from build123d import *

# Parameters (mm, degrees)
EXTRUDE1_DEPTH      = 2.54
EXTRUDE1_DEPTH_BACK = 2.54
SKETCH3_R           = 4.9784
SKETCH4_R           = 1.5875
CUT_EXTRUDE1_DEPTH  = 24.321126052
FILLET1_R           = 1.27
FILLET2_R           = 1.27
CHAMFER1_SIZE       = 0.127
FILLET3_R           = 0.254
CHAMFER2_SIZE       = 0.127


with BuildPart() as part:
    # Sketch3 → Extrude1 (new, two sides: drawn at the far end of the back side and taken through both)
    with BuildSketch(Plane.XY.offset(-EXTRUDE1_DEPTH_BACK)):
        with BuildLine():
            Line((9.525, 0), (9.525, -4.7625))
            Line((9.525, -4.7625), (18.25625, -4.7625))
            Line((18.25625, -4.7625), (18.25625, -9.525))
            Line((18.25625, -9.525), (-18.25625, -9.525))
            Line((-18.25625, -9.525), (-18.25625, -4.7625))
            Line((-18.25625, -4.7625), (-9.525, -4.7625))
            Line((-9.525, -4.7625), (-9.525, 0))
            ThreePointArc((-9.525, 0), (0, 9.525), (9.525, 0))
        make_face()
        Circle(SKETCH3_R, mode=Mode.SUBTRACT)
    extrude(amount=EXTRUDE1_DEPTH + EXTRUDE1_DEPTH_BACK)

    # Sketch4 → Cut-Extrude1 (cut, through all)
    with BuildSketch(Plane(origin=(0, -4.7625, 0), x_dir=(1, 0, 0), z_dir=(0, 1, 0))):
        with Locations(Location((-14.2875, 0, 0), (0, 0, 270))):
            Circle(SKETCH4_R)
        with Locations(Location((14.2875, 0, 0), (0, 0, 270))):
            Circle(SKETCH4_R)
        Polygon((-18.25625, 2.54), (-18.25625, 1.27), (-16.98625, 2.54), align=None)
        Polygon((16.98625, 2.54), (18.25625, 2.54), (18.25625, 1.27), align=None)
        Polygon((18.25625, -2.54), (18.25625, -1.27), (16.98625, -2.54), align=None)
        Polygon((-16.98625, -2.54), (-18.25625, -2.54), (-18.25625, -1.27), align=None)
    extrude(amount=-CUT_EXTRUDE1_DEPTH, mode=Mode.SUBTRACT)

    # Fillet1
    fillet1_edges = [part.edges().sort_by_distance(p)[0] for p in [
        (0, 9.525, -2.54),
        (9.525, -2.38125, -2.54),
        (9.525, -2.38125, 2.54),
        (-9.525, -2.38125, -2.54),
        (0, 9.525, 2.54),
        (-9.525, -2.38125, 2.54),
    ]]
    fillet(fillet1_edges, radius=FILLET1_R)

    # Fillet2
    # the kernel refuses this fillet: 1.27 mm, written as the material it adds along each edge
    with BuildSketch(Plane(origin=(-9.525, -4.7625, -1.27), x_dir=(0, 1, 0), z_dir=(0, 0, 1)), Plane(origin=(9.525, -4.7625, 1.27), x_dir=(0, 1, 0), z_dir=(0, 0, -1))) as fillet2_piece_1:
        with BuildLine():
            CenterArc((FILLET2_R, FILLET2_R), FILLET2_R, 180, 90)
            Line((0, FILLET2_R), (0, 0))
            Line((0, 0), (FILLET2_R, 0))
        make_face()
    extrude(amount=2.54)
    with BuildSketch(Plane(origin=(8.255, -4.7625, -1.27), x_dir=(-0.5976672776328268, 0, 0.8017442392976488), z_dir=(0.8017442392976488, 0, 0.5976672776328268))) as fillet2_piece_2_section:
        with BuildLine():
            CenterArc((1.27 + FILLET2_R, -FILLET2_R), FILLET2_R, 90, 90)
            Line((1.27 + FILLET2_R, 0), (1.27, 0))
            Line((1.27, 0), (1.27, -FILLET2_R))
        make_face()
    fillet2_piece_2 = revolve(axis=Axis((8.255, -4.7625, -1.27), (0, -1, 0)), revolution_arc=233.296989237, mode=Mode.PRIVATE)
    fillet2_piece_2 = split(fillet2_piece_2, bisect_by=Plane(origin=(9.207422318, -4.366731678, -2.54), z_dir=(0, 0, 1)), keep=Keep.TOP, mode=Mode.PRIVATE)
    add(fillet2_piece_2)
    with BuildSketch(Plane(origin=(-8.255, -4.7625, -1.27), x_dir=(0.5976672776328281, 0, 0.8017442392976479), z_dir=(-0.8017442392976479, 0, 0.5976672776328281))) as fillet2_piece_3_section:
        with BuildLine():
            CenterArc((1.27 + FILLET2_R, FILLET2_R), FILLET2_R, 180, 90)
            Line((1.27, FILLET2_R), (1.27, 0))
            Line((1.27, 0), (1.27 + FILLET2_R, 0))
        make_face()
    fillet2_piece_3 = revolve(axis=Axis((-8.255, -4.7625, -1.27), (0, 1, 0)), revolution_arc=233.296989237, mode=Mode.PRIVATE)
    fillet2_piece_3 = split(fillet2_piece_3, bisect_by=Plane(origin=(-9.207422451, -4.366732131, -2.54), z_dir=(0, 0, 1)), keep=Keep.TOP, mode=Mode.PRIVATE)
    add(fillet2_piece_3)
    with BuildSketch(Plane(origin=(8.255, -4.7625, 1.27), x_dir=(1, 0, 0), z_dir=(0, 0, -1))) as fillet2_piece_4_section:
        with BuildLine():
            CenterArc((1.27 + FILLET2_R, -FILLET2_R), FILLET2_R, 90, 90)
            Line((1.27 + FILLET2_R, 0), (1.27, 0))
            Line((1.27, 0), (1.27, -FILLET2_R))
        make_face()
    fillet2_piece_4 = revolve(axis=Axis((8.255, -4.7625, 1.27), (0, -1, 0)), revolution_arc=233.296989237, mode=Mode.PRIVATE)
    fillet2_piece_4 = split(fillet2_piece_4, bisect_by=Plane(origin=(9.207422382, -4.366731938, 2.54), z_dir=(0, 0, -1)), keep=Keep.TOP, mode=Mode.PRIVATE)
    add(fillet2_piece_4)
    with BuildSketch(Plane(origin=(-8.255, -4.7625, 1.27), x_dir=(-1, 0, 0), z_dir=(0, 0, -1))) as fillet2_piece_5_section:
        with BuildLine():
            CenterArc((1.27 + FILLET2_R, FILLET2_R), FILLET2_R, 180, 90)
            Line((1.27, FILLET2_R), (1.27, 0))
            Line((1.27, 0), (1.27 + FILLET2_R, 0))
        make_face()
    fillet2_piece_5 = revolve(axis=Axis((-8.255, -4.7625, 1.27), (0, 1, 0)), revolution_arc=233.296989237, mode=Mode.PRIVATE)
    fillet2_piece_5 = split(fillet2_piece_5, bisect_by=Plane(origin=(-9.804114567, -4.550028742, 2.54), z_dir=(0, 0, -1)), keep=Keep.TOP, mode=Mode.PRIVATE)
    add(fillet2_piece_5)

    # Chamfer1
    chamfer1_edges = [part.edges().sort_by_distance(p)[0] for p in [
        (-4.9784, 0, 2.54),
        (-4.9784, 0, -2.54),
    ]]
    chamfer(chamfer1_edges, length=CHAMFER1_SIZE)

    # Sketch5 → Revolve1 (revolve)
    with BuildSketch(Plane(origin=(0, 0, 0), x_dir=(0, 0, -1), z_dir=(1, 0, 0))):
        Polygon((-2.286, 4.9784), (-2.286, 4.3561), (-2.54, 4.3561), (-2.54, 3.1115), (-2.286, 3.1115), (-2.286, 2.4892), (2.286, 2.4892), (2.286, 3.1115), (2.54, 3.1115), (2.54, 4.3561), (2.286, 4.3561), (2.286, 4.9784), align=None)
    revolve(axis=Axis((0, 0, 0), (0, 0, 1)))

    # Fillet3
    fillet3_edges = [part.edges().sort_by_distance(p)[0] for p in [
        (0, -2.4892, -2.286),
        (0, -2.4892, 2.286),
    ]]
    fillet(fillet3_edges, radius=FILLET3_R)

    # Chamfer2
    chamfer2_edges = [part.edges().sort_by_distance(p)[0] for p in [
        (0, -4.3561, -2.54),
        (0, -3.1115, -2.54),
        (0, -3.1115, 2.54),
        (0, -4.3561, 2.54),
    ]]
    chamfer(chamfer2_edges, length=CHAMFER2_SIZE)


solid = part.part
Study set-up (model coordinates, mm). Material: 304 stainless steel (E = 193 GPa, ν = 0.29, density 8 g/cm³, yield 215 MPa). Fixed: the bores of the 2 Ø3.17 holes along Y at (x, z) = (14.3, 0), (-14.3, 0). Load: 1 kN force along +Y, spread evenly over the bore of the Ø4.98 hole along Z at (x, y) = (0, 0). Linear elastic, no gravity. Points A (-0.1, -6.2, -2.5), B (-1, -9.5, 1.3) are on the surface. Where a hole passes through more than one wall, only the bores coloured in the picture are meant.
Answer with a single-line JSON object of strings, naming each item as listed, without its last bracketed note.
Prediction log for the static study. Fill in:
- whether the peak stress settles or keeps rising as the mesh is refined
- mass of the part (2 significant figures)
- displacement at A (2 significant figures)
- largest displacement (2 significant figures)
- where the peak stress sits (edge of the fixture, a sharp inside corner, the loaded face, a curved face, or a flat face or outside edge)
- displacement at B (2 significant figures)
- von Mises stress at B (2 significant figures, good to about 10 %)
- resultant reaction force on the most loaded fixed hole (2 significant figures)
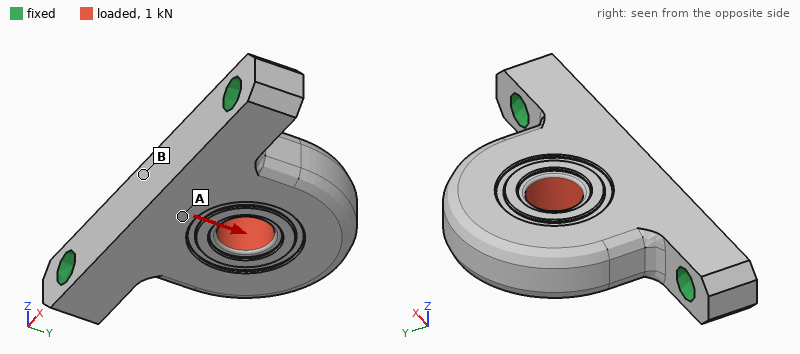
{"whether the peak stress settles or keeps rising as the mesh is refined": "keeps rising", "mass of the part": "15 g", "displacement at A": "3.6 µm", "largest displacement": "3.7 µm", "where the peak stress sits": "edge of the fixture", "displacement at B": "3.5 µm", "von Mises stress at B": "22 MPa", "resultant reaction force on the most loaded fixed hole": "560 N"}
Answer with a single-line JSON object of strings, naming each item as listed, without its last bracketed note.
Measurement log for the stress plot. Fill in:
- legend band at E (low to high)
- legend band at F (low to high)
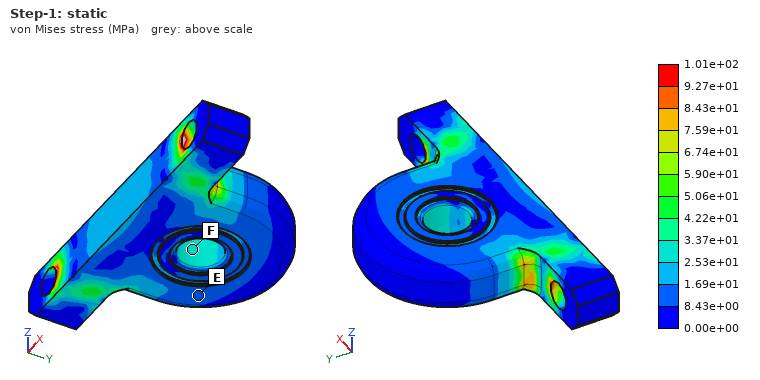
{"legend band at E": "8.43e+00 to 1.69e+01 MPa", "legend band at F": "2.53e+01 to 3.37e+01 MPa"}
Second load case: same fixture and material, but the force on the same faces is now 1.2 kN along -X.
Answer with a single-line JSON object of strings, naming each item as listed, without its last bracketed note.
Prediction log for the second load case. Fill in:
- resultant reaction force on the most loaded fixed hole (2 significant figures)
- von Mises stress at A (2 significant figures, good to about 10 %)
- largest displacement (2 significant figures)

{"resultant reaction force on the most loaded fixed hole": "700 N", "von Mises stress at A": "11 MPa", "largest displacement": "4.1 µm"}
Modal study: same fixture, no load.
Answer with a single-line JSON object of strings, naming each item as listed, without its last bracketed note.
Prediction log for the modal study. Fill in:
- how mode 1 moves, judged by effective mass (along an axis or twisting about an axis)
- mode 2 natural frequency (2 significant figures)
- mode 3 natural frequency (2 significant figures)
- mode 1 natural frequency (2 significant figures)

{"how mode 1 moves, judged by effective mass": "along Z", "mode 2 natural frequency": "27 kHz", "mode 3 natural frequency": "27 kHz", "mode 1 natural frequency": "7700 Hz"}
